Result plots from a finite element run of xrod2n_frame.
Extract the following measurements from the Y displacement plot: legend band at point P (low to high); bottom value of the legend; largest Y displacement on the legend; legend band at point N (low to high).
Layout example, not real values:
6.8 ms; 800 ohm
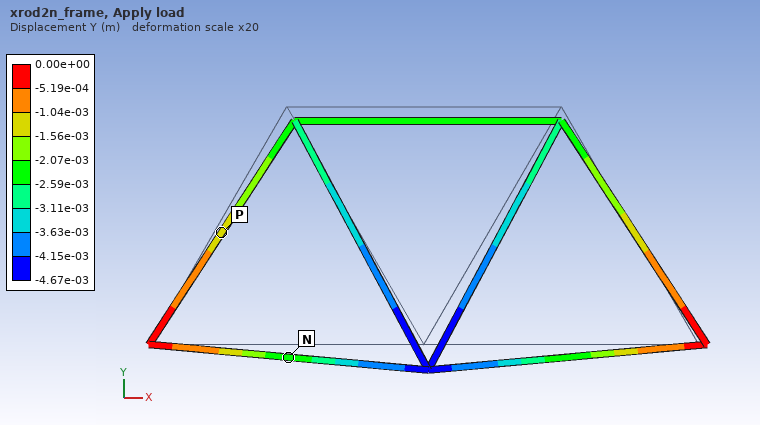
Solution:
-1.56e-03 to -1.04e-03 m; -4.67e-03 m; 0.00e+00 m; -2.59e-03 to -2.07e-03 m
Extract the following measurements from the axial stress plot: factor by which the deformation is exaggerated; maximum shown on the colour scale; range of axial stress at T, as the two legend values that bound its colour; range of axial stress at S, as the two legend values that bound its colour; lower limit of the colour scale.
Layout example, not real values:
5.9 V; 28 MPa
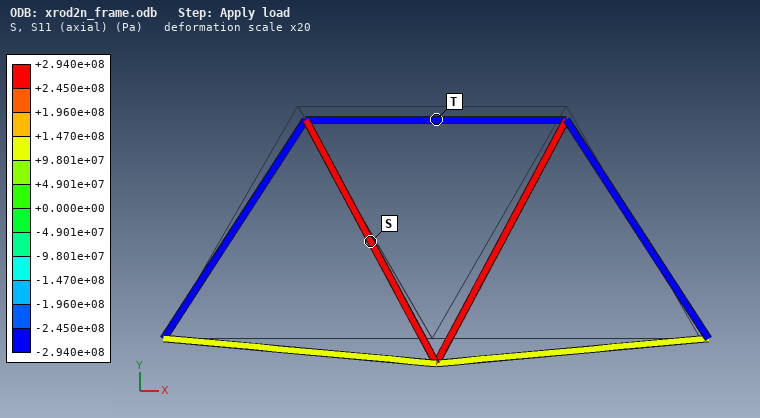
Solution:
20; +2.940e+08 Pa; -2.940e+08 to -2.450e+08 Pa; +2.450e+08 to +2.940e+08 Pa; -2.940e+08 Pa
